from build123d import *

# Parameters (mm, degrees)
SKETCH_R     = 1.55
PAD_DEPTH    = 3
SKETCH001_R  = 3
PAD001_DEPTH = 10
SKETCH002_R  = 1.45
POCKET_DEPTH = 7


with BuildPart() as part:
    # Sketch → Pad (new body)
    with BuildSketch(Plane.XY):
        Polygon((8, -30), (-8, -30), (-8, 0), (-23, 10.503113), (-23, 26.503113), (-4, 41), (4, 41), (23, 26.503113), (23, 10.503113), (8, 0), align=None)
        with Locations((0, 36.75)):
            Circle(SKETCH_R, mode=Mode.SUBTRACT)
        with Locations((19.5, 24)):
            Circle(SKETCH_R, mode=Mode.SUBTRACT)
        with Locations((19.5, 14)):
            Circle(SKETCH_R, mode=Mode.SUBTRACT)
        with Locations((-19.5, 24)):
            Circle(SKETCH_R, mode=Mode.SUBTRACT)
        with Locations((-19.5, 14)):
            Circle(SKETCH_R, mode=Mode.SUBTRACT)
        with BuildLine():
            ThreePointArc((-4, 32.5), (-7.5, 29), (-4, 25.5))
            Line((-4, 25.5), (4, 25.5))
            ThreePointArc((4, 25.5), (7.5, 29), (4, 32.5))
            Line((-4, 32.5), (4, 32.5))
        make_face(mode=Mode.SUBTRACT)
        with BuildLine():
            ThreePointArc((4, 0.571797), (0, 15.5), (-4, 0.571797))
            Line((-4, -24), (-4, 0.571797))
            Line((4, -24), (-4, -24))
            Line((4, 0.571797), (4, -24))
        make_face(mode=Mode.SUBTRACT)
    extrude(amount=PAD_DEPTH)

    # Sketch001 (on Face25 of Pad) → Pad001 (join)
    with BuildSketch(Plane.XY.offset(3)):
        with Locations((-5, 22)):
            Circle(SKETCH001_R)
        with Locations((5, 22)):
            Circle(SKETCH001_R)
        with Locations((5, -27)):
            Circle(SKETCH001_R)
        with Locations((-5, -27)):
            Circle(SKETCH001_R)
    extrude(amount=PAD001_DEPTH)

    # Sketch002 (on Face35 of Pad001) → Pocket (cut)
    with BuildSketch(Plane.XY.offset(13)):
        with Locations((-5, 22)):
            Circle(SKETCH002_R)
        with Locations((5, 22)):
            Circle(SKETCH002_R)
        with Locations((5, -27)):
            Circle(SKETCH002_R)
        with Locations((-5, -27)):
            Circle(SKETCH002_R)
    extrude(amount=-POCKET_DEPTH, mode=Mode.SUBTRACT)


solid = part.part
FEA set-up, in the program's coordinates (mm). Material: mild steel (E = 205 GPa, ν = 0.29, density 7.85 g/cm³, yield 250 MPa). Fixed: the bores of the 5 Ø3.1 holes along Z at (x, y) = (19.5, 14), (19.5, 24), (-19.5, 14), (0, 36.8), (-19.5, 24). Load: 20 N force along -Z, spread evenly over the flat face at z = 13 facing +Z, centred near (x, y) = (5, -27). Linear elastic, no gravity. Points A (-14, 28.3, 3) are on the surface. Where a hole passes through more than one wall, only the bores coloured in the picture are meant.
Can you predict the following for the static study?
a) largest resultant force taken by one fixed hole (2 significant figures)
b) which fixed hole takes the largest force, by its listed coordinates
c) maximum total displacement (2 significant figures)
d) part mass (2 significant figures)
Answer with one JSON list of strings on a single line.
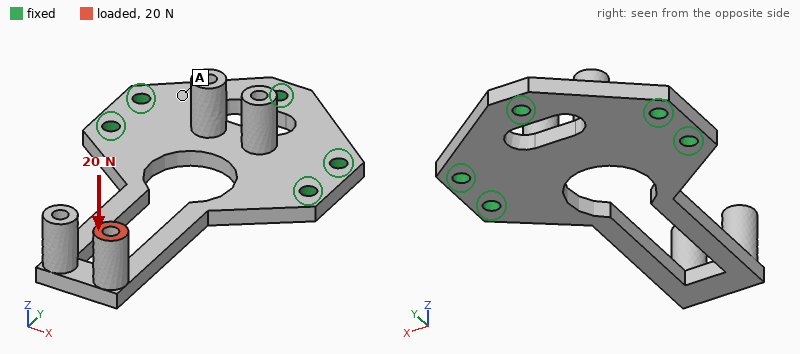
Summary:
["31 N", "(19.5, 14)", "0.13 mm", "41 g"]
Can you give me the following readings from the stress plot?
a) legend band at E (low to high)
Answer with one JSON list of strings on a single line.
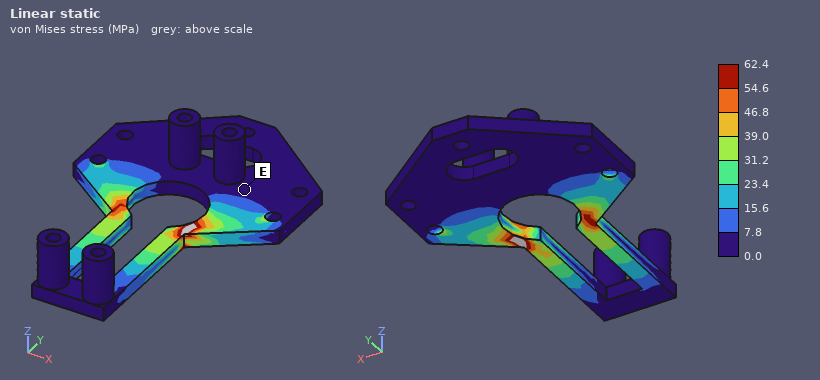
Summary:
["0.0 to 7.8 MPa"]
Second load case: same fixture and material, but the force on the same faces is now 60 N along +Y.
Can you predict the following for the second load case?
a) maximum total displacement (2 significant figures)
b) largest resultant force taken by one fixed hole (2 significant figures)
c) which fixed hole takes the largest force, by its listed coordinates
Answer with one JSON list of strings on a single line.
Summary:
["0.18 mm", "32 N", "(19.5, 24)"]
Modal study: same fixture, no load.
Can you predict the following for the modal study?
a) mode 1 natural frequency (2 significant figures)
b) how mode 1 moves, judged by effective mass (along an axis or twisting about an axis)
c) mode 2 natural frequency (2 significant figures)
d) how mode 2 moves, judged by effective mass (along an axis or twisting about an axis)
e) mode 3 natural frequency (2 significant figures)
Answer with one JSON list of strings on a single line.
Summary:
["810 Hz", "along Z", "2400 Hz", "along X", "3800 Hz"]
